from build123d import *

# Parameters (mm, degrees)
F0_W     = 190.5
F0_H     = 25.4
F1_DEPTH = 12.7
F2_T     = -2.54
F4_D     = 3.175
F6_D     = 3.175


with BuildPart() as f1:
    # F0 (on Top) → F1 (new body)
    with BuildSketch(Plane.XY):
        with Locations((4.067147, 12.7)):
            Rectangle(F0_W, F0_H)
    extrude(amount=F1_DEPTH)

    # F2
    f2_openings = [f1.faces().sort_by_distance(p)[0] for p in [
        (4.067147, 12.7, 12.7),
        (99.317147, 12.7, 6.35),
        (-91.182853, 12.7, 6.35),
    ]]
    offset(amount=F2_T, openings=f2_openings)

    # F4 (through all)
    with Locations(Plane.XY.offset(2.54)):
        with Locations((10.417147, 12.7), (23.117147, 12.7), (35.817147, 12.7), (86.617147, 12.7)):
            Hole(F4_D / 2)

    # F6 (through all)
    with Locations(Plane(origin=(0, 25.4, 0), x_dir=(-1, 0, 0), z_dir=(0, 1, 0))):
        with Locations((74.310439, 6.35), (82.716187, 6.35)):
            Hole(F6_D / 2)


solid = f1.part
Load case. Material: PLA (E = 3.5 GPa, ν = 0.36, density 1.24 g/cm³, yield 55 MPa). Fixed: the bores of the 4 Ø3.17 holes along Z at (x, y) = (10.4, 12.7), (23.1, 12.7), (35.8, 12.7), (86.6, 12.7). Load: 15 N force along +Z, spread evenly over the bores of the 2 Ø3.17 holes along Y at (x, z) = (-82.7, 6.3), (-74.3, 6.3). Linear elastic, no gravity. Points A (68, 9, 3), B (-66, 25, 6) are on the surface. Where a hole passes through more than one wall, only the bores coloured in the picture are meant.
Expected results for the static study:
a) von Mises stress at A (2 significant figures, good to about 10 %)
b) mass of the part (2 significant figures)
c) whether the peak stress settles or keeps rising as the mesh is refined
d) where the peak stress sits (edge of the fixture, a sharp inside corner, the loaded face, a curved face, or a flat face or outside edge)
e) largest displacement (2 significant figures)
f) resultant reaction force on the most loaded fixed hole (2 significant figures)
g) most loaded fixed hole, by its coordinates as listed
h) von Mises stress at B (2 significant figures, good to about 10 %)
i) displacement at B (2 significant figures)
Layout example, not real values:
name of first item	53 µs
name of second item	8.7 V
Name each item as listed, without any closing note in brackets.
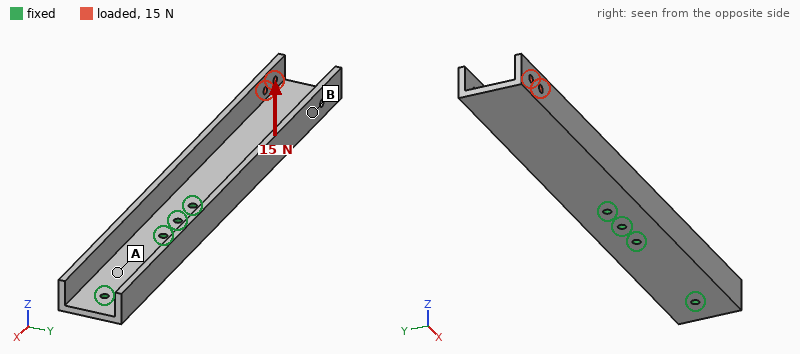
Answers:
von Mises stress at A	0.82 MPa
mass of the part	27 g
whether the peak stress settles or keeps rising as the mesh is refined	keeps rising
where the peak stress sits	edge of the fixture
largest displacement	1.8 mm
resultant reaction force on the most loaded fixed hole	78 N
most loaded fixed hole, by its coordinates as listed	(10.4, 12.7)
von Mises stress at B	1.6 MPa
displacement at B	0.52 mm
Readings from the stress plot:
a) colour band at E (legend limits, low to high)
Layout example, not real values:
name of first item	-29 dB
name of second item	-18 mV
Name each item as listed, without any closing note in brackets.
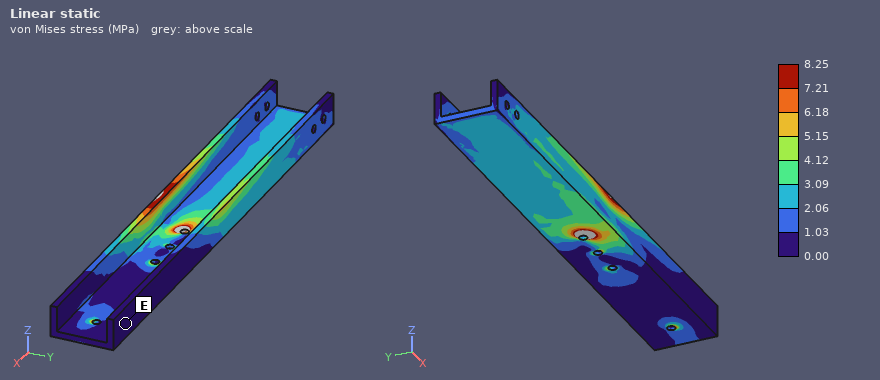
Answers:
colour band at E	0.00 to 1.03 MPa
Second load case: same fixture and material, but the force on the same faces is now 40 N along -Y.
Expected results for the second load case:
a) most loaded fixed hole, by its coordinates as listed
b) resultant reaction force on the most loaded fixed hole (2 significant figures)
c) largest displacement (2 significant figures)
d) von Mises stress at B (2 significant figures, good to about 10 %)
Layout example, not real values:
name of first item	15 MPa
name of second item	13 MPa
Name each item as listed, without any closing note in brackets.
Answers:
most loaded fixed hole, by its coordinates as listed	(10.4, 12.7)
resultant reaction force on the most loaded fixed hole	160 N
largest displacement	1.9 mm
von Mises stress at B	3.3 MPa
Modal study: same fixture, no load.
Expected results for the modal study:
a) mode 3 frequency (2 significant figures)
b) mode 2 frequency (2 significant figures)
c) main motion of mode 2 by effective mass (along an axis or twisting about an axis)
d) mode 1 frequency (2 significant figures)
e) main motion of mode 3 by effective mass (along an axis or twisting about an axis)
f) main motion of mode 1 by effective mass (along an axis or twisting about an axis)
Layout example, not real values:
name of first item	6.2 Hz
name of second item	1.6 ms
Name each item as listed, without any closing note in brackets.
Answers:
mode 3 frequency	630 Hz
mode 2 frequency	360 Hz
main motion of mode 2 by effective mass	along Y
mode 1 frequency	250 Hz
main motion of mode 3 by effective mass	along Y
main motion of mode 1 by effective mass	along Z
